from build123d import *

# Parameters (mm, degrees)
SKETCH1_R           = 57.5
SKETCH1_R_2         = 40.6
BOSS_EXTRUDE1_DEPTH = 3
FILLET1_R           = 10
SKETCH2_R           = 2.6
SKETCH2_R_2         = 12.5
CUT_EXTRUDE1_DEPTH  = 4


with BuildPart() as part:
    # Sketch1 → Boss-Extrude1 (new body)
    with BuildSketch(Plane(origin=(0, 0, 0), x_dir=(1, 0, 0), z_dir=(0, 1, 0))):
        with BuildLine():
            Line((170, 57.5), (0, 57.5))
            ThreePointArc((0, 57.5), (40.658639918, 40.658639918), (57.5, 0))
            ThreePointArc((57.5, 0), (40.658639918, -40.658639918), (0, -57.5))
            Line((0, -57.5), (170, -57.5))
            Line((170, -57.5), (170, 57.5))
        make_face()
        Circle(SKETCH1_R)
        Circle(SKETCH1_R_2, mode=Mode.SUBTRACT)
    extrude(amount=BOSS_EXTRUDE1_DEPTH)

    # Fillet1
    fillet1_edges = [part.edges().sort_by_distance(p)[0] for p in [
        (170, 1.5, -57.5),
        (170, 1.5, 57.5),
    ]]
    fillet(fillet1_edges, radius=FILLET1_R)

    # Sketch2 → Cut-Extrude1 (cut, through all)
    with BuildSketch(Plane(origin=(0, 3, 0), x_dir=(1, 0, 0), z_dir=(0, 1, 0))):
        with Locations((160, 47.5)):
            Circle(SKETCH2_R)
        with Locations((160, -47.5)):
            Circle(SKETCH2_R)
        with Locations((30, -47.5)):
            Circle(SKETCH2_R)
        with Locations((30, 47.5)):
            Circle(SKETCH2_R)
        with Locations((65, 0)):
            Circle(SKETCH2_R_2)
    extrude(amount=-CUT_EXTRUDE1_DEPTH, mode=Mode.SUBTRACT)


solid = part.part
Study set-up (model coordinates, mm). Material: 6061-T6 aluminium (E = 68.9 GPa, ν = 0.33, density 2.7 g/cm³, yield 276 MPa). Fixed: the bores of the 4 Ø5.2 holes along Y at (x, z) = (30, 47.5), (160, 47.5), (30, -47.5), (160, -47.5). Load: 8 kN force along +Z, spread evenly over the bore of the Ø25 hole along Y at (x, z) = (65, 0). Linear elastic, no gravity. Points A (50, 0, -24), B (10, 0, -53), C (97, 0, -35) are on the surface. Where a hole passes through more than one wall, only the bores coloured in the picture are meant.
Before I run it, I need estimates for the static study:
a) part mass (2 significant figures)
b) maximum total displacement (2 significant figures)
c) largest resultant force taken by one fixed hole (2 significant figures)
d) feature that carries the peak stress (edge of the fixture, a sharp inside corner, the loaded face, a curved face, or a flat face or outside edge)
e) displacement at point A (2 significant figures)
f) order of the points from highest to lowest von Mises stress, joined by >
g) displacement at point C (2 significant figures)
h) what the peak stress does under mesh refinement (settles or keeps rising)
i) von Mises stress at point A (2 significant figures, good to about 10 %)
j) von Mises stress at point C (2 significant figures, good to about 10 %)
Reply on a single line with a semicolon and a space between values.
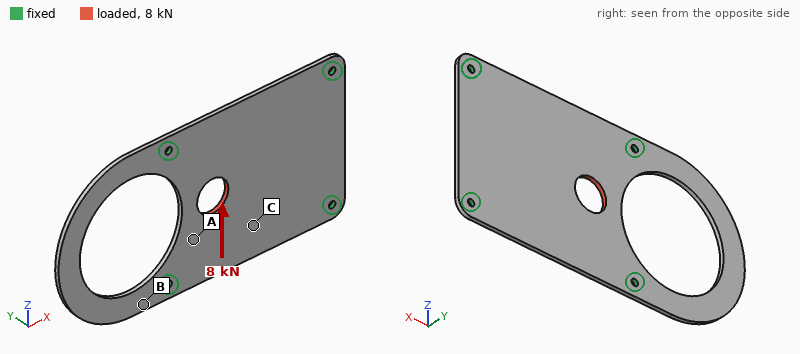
150 g; 50 µm; 2.8 kN; edge of the fixture; 33 µm; A > C > B; 35 µm; keeps rising; 29 MPa; 18 MPa
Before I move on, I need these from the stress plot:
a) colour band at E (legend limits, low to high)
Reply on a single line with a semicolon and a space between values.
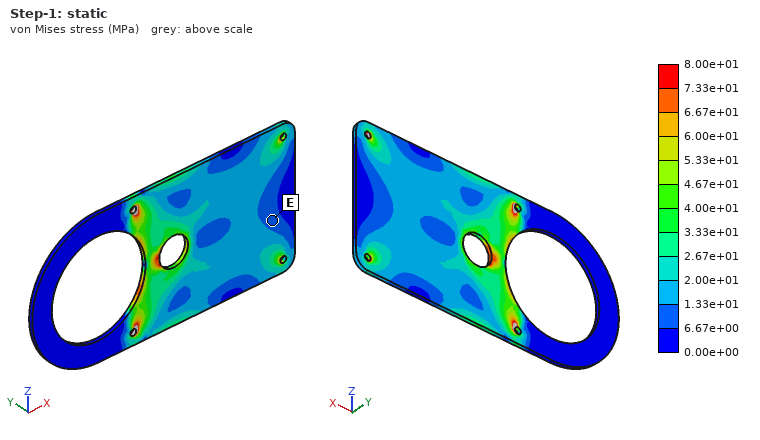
6.67e+00 to 1.33e+01 MPa
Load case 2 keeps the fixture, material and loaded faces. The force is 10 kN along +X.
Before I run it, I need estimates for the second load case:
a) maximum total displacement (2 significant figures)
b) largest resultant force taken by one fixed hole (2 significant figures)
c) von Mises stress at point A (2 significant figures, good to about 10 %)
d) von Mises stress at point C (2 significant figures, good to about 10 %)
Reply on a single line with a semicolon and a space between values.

64 µm; 3.4 kN; 30 MPa; 21 MPa
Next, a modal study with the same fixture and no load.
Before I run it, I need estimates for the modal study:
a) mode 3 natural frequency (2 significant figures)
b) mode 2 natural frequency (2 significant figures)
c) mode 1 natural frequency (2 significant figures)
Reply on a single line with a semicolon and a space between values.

760 Hz; 740 Hz; 280 Hz
